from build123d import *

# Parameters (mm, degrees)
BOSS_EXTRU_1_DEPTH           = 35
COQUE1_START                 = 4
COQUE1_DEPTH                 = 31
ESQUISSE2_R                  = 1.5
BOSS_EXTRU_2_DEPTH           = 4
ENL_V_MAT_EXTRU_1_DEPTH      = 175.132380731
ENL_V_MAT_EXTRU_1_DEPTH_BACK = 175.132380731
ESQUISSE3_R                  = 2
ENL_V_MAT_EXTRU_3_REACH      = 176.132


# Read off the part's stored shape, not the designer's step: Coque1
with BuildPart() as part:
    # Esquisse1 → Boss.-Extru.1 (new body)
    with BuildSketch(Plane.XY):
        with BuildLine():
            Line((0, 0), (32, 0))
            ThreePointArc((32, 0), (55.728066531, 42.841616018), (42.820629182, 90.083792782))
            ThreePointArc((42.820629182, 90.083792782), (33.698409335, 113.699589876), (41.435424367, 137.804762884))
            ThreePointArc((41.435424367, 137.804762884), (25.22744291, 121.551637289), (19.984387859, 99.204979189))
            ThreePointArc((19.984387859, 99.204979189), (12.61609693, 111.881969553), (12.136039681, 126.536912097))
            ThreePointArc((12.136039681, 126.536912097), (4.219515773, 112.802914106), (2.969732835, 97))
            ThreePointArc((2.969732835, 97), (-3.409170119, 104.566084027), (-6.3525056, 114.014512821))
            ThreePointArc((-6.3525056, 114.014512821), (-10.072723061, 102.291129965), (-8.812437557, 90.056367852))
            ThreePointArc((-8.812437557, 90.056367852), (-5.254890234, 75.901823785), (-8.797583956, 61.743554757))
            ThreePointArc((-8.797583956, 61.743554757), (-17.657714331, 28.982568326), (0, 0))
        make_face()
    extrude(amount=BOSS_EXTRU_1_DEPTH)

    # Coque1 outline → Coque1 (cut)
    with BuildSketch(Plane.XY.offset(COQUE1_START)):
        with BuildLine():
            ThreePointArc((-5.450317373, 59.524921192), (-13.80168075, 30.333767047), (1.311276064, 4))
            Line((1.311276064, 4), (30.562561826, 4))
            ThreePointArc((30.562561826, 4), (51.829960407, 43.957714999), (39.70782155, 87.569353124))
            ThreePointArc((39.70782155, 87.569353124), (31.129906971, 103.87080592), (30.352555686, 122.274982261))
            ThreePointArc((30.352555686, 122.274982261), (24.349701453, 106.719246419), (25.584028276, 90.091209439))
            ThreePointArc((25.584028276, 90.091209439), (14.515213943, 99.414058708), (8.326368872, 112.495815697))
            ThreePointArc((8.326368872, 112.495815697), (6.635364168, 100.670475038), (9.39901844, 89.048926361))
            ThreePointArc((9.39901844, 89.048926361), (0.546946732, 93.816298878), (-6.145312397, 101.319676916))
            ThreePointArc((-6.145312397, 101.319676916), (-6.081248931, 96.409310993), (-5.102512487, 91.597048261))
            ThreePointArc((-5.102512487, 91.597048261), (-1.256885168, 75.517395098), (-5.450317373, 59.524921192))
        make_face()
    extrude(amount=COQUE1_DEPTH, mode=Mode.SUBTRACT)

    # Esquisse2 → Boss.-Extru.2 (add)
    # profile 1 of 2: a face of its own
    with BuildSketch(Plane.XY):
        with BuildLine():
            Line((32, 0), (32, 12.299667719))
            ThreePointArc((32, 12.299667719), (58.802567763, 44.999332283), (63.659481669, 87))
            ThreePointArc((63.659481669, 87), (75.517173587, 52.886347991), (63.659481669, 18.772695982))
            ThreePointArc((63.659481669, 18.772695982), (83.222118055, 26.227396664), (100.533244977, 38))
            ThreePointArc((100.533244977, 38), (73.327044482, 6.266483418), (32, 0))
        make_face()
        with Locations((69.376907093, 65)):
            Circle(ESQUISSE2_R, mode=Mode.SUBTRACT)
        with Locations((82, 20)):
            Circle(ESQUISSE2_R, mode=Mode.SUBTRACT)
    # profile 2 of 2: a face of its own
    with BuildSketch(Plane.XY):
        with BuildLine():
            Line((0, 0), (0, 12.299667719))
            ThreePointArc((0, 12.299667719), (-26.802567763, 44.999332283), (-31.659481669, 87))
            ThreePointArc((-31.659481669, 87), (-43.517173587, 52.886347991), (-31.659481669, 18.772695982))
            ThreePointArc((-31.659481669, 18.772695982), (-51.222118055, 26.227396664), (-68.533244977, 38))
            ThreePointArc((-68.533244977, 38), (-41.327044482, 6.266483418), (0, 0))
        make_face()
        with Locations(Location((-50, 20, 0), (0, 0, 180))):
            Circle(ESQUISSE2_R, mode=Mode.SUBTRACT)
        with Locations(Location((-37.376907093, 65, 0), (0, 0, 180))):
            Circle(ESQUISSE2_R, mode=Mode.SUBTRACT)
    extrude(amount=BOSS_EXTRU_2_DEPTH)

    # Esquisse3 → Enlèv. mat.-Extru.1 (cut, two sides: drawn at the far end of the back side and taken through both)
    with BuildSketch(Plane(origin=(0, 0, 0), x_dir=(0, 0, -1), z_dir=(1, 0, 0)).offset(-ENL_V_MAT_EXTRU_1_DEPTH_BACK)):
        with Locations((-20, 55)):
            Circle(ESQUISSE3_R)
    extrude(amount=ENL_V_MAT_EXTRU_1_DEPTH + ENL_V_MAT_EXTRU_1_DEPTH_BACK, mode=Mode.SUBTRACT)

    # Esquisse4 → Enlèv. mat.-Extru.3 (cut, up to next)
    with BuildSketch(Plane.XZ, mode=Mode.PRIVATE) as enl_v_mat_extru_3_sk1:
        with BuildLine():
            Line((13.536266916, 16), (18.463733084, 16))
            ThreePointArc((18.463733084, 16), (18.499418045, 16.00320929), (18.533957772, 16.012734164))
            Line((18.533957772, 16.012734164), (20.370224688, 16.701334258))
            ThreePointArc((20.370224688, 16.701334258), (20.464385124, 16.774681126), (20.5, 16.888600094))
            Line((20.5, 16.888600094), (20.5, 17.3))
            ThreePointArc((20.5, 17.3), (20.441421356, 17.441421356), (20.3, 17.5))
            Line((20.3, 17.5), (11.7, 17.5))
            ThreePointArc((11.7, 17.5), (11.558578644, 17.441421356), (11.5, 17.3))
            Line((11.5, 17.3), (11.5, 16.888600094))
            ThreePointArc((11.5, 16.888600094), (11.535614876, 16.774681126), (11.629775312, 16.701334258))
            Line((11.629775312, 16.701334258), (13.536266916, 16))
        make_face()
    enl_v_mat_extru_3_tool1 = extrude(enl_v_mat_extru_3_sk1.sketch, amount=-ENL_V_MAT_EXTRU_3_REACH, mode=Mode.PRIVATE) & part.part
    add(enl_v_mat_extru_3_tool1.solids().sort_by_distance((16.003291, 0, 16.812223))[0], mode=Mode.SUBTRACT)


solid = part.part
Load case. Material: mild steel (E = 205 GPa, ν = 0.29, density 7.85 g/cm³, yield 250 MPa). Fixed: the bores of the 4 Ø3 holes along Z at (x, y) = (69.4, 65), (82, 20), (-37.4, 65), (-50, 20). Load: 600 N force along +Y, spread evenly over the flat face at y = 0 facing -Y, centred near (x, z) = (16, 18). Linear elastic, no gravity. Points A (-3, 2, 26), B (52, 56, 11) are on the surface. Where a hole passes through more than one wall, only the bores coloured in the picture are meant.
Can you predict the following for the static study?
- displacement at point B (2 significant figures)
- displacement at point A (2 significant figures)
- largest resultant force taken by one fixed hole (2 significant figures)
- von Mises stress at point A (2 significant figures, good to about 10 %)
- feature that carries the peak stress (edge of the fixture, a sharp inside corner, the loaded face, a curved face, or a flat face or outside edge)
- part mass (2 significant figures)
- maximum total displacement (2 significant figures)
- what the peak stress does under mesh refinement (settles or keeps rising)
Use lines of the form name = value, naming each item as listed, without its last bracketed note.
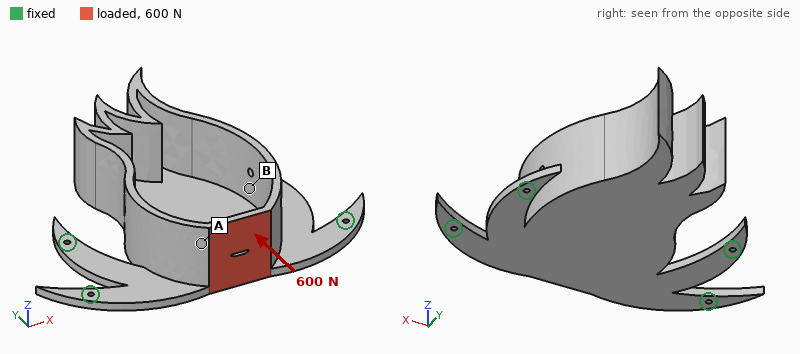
displacement at point B = 0.052 mm
displacement at point A = 0.076 mm
largest resultant force taken by one fixed hole = 300 N
von Mises stress at point A = 9.6 MPa
feature that carries the peak stress = edge of the fixture
part mass = 710 g
maximum total displacement = 0.21 mm
what the peak stress does under mesh refinement = keeps rising
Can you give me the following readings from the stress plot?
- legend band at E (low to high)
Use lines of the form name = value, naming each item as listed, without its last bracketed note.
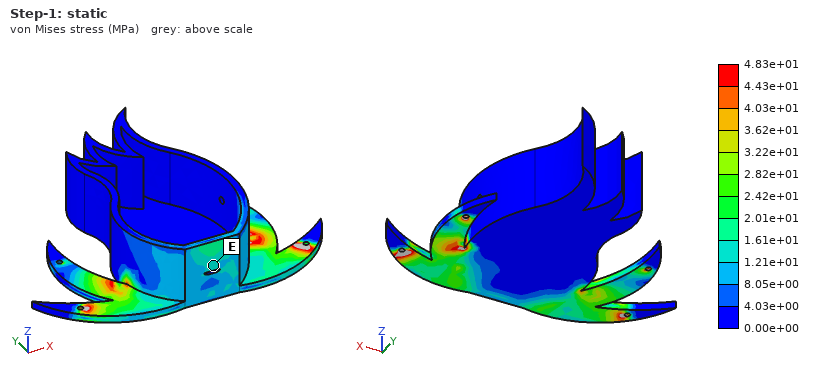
legend band at E = 1.21e+01 to 1.61e+01 MPa
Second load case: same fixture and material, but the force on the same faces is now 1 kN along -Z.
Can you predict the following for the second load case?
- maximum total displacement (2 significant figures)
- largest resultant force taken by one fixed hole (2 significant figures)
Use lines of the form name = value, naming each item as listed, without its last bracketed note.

maximum total displacement = 0.55 mm
largest resultant force taken by one fixed hole = 680 N
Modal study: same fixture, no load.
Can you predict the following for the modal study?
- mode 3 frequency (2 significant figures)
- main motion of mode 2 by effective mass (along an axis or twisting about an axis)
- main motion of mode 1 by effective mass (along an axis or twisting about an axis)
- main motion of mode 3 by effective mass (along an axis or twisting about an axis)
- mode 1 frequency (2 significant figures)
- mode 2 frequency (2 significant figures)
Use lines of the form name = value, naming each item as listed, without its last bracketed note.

mode 3 frequency = 1100 Hz
main motion of mode 2 by effective mass = along Z
main motion of mode 1 by effective mass = along Z
main motion of mode 3 by effective mass = along X
mode 1 frequency = 230 Hz
mode 2 frequency = 870 Hz
